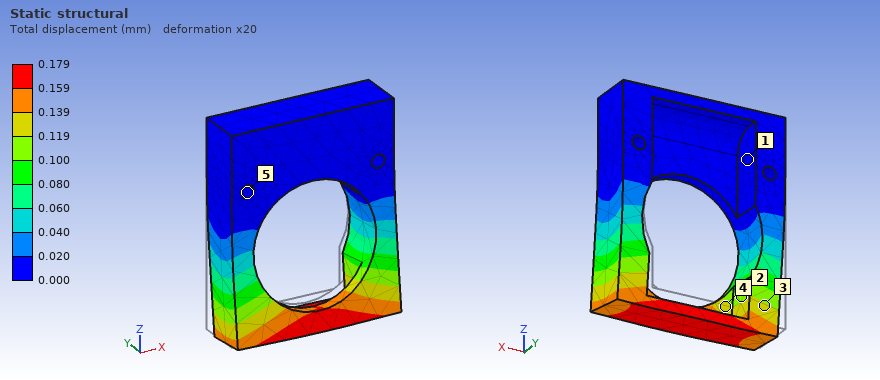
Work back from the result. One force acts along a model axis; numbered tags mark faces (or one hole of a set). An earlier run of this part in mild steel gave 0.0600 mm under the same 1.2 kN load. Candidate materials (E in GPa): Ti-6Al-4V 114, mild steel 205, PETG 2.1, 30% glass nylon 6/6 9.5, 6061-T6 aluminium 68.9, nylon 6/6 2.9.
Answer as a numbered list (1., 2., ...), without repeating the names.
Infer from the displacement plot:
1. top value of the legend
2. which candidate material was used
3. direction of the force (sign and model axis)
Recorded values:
1. 0.179 mm
2. 6061-T6 aluminium
3. -Y
